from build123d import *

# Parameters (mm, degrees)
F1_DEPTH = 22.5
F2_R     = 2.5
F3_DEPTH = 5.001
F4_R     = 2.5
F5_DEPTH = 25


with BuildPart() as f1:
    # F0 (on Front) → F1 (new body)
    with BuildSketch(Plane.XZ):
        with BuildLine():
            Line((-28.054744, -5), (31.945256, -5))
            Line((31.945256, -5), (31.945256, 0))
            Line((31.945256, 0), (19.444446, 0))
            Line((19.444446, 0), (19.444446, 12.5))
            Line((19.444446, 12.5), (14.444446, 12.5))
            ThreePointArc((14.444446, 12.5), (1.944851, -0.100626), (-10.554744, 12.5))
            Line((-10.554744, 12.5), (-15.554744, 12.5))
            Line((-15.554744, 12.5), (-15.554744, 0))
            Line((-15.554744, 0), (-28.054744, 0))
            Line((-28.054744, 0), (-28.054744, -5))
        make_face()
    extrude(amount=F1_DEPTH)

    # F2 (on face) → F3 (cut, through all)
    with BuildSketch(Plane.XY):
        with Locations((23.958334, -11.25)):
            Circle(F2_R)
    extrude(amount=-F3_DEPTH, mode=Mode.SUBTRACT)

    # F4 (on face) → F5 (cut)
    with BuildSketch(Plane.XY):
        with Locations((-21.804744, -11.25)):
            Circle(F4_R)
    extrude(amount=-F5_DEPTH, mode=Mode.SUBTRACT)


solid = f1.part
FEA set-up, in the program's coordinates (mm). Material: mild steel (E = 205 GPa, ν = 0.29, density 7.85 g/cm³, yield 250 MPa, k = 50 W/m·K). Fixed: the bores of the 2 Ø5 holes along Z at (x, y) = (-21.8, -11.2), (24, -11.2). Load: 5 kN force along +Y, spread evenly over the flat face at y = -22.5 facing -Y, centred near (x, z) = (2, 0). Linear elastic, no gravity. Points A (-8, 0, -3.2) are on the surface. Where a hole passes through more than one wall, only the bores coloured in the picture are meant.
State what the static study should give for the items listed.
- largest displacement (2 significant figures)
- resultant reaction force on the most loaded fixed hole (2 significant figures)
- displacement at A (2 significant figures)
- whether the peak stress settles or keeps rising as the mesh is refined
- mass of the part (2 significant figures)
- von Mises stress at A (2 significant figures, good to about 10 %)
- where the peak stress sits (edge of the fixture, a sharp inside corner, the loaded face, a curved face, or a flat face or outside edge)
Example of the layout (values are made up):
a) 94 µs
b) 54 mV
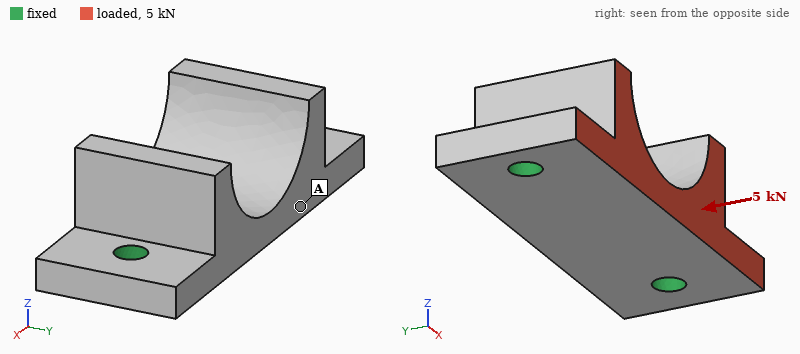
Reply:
a) 16 µm
b) 2.6 kN
c) 7.9 µm
d) keeps rising
e) 85 g
f) 30 MPa
g) edge of the fixture
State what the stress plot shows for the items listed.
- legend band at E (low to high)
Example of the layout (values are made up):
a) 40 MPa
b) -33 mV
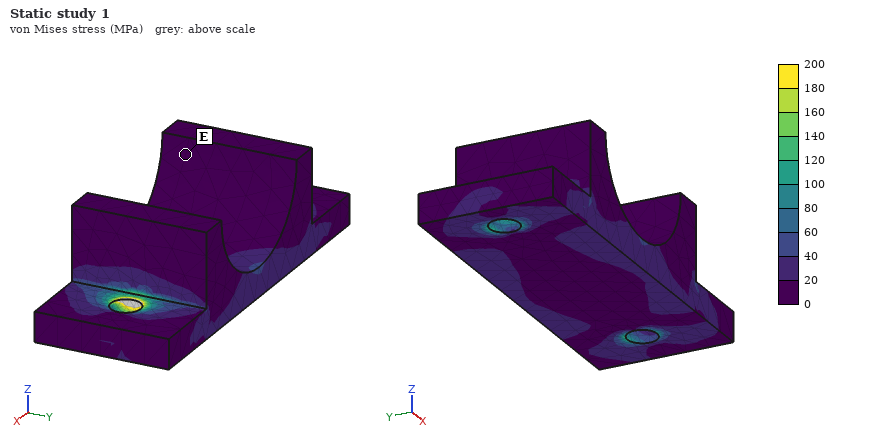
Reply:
a) 0 to 20 MPa
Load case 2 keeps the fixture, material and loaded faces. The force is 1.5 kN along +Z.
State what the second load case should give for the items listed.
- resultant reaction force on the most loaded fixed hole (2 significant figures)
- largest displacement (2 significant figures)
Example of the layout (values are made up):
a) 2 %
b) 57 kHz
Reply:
a) 800 N
b) 16 µm
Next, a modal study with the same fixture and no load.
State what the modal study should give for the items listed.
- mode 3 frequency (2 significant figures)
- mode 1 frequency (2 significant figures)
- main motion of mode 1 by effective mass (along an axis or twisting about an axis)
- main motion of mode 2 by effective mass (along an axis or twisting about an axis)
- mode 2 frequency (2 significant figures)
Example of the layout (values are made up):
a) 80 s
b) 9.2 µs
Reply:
a) 17 kHz
b) 9100 Hz
c) along Z
d) along Y
e) 10 kHz
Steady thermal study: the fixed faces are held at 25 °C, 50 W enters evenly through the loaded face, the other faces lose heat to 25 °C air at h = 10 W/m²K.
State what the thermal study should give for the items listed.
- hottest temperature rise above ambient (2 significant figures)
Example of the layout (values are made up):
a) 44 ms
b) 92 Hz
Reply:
a) 56 K
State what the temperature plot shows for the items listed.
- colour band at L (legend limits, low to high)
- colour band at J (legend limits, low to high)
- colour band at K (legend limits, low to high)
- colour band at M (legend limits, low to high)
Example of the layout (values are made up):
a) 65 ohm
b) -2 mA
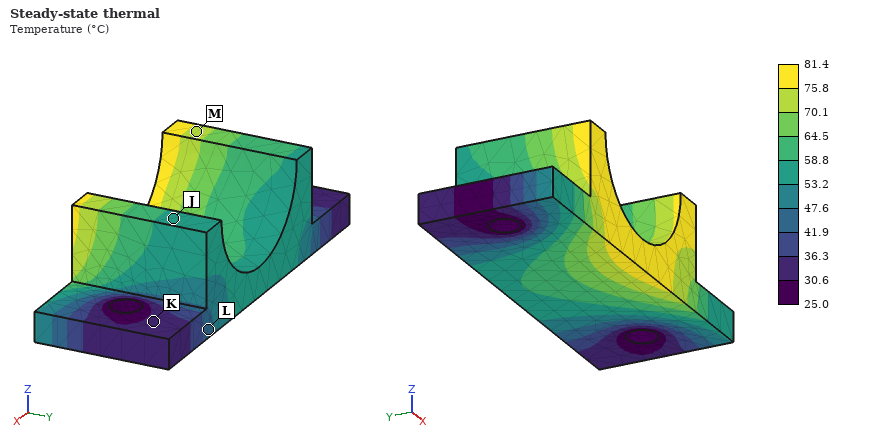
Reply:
a) 41.9 to 47.6 °C
b) 53.2 to 58.8 °C
c) 30.6 to 36.3 °C
d) 70.1 to 75.8 °C
